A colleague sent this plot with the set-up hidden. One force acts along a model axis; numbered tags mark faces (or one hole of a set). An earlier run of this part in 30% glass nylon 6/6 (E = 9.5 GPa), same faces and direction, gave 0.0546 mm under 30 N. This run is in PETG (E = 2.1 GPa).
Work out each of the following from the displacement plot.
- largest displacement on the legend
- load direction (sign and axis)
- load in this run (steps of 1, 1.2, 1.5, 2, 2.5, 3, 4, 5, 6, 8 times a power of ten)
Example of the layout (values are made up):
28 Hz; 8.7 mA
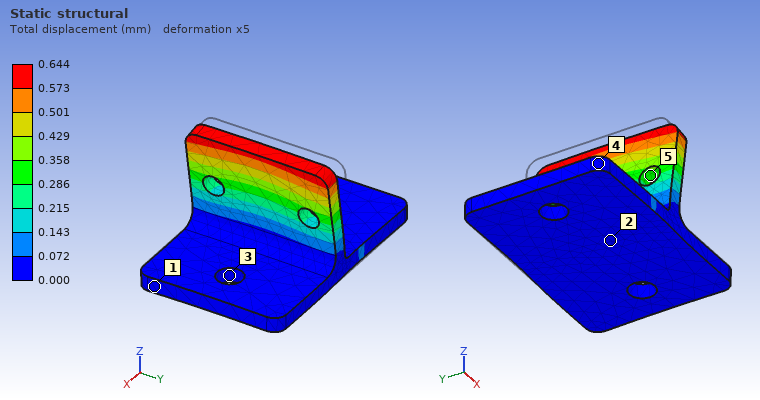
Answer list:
0.644 mm; +X; 80 N
